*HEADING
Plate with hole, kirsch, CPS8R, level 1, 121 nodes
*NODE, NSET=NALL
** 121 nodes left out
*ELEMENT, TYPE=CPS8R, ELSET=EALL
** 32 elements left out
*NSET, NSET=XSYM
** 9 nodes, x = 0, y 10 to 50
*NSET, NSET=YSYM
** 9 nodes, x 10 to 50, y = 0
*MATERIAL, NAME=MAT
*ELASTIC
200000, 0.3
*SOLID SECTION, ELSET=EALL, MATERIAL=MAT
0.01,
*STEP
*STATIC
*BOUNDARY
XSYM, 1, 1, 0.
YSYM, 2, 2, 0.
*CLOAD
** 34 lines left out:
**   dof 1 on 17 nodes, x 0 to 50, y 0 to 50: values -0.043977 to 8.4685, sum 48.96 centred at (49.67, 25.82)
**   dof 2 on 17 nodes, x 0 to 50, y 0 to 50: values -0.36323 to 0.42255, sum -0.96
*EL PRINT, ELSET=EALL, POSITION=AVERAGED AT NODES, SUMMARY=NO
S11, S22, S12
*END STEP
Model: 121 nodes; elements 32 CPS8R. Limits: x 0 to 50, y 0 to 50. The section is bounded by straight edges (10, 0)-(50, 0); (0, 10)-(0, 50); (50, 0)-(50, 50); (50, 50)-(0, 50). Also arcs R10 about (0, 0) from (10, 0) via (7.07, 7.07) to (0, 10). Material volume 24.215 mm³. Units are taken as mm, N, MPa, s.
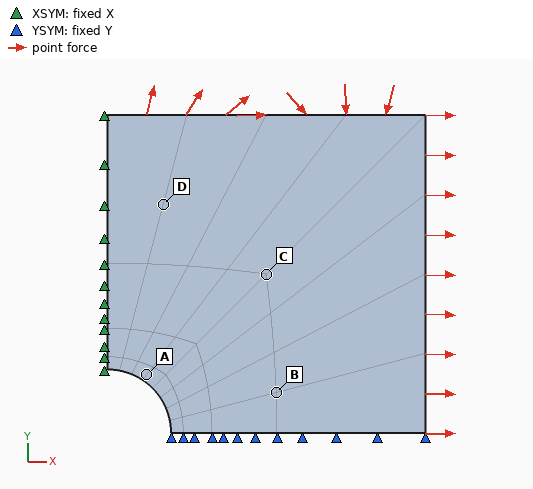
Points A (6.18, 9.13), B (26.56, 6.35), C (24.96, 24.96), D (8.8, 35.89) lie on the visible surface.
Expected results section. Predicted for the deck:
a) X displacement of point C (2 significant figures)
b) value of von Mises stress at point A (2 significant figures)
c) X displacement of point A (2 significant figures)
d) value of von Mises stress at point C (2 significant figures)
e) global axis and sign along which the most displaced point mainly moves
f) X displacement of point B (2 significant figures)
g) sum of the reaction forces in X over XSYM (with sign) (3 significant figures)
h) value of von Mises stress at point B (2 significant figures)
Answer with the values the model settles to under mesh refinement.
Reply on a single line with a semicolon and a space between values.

0.014 mm; 150 MPa; 0.0077 mm; 110 MPa; +X; 0.018 mm; -49.0 N; 81 MPa
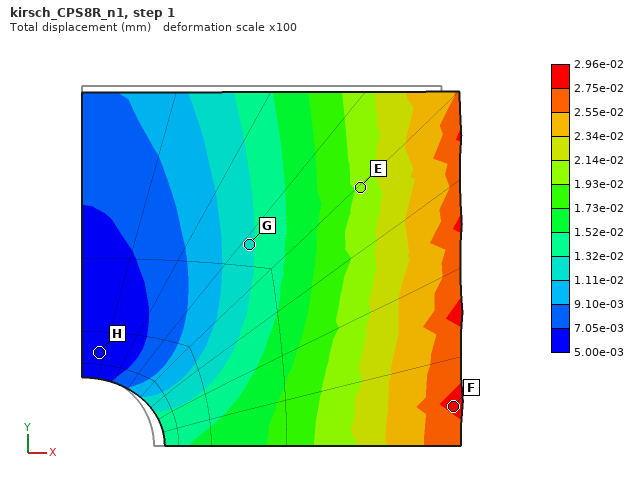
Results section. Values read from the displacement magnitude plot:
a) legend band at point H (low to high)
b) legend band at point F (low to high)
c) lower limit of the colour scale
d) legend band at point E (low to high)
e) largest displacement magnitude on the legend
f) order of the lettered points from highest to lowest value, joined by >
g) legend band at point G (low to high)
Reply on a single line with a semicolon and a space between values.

5.00e-03 to 7.05e-03 mm; 2.75e-02 to 2.96e-02 mm; 5.00e-03 mm; 1.93e-02 to 2.14e-02 mm; 2.96e-02 mm; F > E > G > H; 1.11e-02 to 1.32e-02 mm
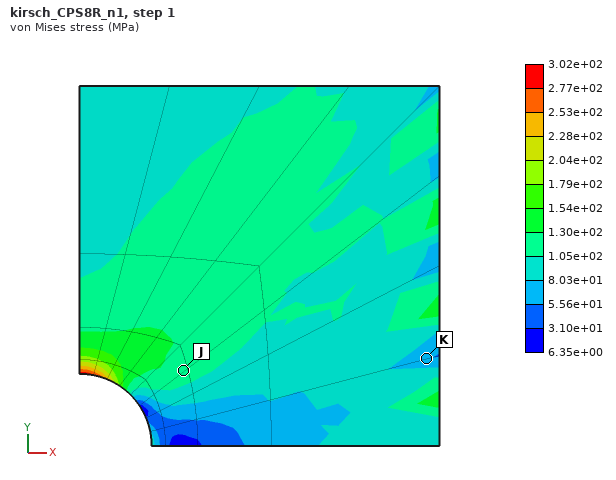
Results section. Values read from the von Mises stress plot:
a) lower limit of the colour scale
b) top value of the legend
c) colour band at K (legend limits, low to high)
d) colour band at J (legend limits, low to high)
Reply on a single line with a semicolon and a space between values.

6.35e+00 MPa; 3.02e+02 MPa; 5.56e+01 to 8.03e+01 MPa; 1.05e+02 to 1.30e+02 MPa
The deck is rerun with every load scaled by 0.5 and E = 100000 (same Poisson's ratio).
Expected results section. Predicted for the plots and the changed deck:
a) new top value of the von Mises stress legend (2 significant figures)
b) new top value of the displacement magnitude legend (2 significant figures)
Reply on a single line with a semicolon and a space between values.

150 MPa; 0.030 mm
